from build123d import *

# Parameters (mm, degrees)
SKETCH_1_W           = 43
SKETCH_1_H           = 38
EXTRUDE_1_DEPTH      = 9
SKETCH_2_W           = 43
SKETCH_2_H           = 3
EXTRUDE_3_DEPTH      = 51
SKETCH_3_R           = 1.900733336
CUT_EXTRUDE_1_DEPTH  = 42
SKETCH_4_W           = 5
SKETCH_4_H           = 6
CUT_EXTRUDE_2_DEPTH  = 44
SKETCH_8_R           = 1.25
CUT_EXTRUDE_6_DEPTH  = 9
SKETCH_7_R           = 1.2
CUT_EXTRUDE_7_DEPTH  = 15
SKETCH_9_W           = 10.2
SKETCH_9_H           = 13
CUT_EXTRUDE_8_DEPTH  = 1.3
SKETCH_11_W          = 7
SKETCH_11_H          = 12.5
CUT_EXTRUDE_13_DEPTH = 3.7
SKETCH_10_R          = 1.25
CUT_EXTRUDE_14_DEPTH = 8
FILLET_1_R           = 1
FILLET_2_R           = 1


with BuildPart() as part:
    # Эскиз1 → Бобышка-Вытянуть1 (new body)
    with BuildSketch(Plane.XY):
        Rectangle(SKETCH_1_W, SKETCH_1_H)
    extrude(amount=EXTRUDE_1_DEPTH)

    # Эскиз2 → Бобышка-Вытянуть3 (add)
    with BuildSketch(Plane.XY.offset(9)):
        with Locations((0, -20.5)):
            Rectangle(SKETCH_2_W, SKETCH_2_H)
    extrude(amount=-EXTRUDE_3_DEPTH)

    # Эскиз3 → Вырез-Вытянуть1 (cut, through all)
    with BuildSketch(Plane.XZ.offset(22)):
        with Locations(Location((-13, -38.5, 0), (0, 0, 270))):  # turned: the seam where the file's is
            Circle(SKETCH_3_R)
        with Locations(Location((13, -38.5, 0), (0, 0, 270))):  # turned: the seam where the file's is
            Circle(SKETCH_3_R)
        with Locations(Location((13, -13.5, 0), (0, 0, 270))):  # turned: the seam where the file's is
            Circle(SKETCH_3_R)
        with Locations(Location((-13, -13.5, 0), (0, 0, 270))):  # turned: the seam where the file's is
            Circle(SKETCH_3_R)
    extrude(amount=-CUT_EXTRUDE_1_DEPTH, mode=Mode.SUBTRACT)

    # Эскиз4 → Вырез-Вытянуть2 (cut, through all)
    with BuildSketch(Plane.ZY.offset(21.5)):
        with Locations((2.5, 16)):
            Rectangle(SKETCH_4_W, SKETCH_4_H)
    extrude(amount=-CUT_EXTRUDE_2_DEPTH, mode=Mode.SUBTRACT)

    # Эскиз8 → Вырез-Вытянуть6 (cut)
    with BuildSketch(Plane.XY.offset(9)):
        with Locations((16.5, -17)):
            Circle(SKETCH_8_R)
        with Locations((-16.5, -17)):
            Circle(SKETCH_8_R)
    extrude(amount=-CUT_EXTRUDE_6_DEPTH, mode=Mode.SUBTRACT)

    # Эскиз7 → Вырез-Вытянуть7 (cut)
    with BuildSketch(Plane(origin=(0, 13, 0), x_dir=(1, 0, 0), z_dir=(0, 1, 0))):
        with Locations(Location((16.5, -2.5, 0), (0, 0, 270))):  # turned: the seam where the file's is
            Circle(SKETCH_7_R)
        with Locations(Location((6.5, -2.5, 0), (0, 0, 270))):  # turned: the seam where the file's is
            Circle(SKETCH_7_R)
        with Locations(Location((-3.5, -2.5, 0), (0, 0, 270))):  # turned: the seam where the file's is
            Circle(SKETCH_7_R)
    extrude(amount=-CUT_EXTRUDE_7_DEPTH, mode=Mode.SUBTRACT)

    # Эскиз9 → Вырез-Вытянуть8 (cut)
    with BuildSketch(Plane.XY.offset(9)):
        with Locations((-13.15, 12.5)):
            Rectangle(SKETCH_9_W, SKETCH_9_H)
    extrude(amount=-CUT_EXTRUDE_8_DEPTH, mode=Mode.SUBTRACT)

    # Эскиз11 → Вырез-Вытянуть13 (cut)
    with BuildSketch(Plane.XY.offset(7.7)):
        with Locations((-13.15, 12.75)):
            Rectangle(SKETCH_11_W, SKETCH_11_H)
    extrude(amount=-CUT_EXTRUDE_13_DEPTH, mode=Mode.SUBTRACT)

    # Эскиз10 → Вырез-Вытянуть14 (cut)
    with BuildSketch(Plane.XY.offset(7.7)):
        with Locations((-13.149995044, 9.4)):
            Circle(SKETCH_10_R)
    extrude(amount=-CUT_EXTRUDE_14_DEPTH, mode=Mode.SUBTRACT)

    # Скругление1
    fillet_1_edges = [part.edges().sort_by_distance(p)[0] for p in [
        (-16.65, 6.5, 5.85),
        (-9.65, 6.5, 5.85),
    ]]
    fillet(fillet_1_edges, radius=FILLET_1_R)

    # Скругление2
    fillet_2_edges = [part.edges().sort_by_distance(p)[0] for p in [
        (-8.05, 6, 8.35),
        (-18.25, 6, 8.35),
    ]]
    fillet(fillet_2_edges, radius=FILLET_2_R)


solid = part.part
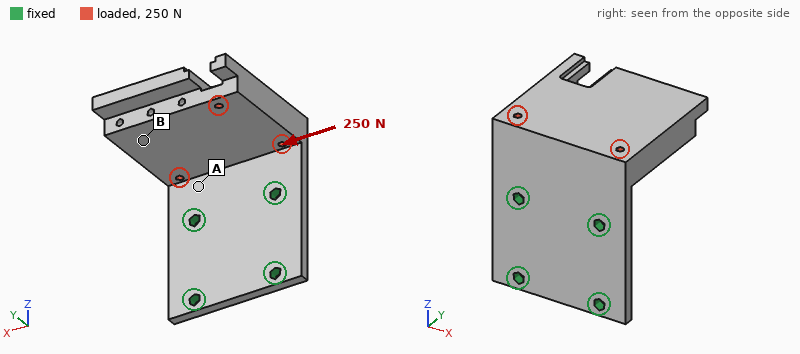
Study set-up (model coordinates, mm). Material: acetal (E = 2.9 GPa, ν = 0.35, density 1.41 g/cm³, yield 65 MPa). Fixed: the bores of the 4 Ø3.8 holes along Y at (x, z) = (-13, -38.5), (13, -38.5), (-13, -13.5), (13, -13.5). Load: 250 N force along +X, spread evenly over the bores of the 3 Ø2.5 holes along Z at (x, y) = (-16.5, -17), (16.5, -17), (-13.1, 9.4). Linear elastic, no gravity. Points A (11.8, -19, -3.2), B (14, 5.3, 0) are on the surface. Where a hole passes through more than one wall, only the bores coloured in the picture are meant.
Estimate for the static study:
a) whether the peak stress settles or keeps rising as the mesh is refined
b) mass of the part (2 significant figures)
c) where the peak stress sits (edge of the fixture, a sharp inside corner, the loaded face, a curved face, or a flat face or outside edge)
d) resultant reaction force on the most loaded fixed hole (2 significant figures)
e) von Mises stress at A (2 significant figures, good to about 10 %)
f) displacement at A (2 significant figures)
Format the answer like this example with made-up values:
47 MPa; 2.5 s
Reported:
keeps rising; 27 g; edge of the fixture; 200 N; 12 MPa; 0.12 mm
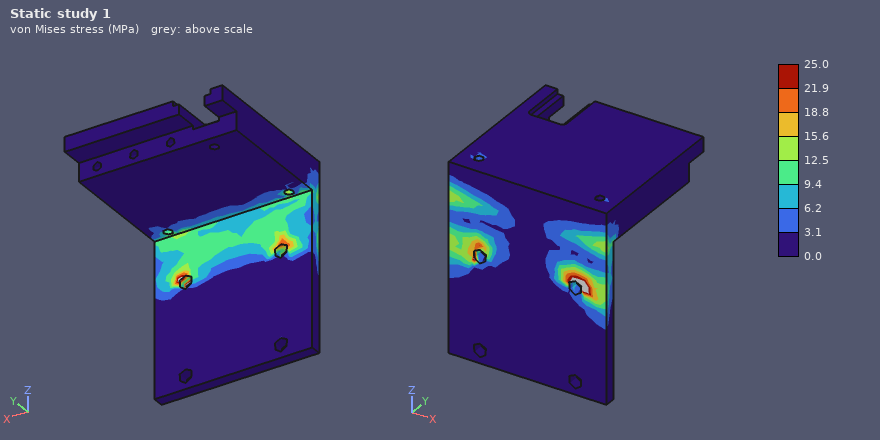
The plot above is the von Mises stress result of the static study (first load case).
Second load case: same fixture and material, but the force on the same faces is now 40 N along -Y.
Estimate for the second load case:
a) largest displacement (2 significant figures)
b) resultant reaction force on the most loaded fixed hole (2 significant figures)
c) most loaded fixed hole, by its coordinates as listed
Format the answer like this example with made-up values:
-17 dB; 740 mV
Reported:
0.86 mm; 26 N; (-13, -13.5)
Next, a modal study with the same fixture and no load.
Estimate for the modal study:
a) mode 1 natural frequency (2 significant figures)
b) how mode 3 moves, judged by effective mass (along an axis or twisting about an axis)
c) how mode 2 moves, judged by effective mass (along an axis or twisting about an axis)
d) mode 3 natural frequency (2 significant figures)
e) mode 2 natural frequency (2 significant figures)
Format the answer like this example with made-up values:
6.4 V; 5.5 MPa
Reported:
220 Hz; along Y; along X; 1200 Hz; 590 Hz
